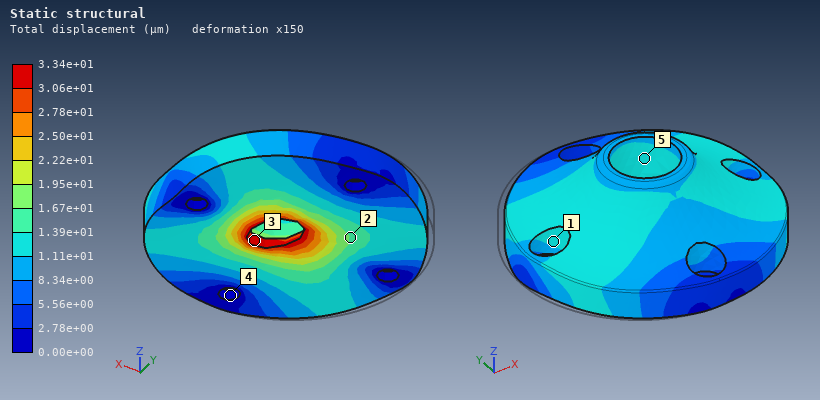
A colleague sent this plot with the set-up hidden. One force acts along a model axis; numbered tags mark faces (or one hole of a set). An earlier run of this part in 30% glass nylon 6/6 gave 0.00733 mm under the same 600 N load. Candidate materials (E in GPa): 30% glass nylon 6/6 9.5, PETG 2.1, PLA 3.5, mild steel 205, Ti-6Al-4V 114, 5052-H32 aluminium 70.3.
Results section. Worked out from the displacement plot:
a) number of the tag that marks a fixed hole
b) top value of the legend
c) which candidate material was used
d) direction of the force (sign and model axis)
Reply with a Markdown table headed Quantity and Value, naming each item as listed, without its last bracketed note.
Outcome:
| Quantity | Value |
|---|---|
| number of the tag that marks a fixed hole | 4 |
| top value of the legend | 3.34e+01 µm |
| which candidate material was used | PETG |
| direction of the force | +X |
